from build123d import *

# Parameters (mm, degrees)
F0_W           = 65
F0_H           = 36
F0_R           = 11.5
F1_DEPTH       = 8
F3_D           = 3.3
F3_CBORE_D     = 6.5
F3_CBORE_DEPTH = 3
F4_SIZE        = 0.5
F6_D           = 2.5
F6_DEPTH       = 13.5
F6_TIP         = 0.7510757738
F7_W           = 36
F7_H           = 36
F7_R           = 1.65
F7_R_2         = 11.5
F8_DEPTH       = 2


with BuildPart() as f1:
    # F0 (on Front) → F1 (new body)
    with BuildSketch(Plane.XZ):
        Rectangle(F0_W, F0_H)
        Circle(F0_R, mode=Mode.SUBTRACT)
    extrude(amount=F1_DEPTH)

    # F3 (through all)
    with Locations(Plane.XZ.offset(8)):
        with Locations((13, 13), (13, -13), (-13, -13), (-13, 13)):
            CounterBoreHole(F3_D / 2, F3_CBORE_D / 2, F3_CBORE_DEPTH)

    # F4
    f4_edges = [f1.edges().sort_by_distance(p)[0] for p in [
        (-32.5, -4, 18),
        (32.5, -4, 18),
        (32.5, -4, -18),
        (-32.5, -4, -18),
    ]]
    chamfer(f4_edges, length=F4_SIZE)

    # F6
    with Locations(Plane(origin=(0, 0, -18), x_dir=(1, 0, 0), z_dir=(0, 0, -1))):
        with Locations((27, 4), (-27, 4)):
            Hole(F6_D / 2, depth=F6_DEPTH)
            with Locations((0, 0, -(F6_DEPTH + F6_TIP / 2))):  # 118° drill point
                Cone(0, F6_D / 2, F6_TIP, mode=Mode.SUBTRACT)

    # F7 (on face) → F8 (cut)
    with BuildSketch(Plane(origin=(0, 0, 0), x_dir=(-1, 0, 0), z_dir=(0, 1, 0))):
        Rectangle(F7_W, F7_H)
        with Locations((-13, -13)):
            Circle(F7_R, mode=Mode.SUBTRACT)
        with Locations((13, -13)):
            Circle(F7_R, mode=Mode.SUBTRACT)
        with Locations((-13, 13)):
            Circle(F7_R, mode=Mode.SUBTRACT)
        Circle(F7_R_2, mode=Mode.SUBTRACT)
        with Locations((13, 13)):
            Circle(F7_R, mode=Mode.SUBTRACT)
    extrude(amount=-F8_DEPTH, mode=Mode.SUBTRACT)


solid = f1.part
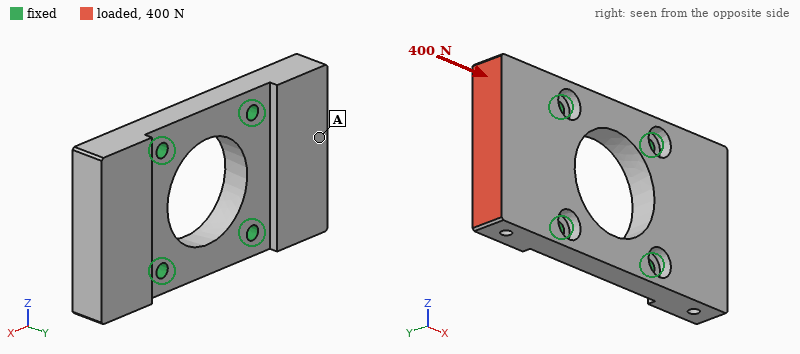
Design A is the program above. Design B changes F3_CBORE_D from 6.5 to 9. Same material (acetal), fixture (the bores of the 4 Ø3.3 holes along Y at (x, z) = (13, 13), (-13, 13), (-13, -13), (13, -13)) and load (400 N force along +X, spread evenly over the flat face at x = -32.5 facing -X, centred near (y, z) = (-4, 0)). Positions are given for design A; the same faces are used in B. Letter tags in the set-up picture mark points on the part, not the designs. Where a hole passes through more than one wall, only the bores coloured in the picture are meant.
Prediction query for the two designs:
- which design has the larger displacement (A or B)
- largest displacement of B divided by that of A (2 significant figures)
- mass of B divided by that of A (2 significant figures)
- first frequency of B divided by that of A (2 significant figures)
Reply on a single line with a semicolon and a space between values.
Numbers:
B; 1.3; 0.97; 0.90
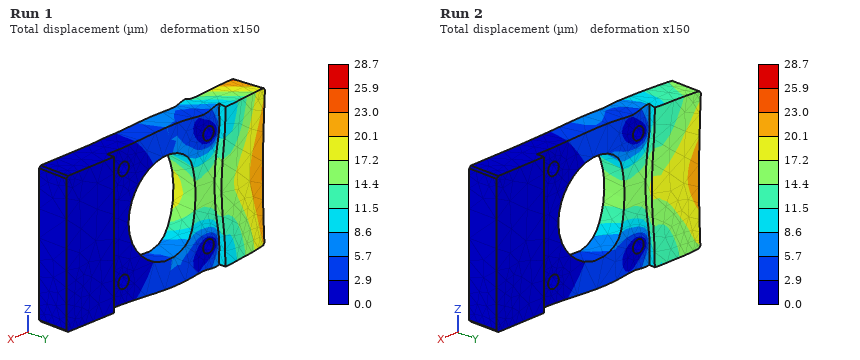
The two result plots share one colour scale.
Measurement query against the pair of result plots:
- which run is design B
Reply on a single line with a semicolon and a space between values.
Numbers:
Run 1
